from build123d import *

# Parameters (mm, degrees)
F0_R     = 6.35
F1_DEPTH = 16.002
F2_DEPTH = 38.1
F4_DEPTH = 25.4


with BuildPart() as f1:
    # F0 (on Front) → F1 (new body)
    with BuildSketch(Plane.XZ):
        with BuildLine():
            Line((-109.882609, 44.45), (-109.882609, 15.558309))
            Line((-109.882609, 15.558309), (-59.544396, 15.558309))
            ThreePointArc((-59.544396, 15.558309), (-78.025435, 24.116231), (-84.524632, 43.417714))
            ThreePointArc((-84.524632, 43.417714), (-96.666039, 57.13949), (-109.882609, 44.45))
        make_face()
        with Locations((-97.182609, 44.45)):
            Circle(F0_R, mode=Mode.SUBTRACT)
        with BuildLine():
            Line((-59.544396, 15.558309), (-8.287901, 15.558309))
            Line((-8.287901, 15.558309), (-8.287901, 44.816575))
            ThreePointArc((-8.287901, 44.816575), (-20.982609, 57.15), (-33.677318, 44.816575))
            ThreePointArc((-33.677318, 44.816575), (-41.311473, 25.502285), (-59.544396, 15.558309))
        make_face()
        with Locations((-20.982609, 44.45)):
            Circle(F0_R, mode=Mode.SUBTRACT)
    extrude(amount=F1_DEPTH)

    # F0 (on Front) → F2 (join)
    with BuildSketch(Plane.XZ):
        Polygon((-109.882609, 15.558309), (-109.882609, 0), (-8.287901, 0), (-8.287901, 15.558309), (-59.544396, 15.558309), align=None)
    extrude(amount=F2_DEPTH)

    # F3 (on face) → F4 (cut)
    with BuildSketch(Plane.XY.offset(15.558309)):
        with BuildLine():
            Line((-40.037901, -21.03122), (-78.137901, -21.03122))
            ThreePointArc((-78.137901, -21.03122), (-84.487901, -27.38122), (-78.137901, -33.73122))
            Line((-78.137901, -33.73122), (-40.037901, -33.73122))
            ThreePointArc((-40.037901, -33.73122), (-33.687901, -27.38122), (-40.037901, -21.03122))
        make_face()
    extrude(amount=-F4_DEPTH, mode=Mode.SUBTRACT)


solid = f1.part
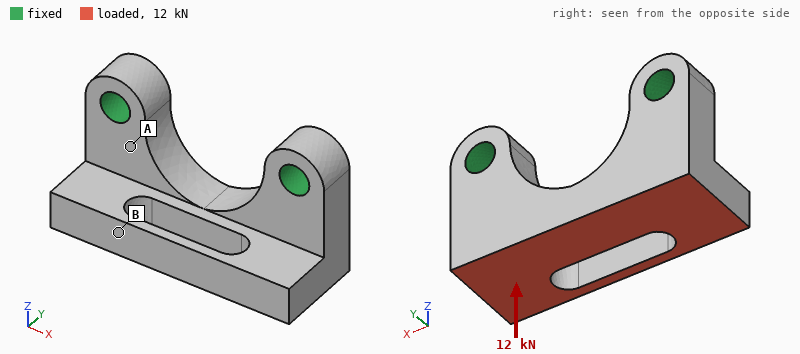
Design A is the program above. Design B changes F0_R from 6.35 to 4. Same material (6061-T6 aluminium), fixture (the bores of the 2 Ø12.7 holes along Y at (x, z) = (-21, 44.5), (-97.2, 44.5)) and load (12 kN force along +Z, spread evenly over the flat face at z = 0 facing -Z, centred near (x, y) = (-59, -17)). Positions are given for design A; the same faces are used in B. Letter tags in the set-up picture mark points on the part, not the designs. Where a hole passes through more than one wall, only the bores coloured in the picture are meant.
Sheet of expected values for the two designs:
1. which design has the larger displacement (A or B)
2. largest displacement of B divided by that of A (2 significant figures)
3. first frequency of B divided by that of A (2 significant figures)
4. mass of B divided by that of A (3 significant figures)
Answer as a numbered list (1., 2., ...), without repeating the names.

1. B
2. 1.1
3. 0.88
4. 1.03
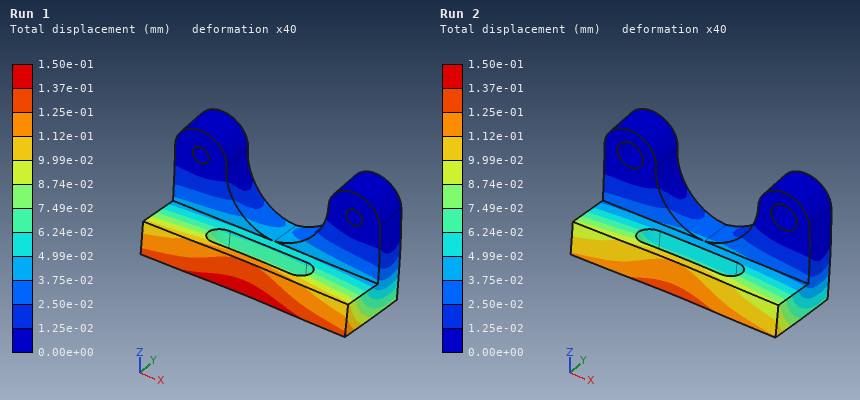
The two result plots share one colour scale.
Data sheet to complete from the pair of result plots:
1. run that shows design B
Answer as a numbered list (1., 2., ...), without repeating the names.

1. Run 1
